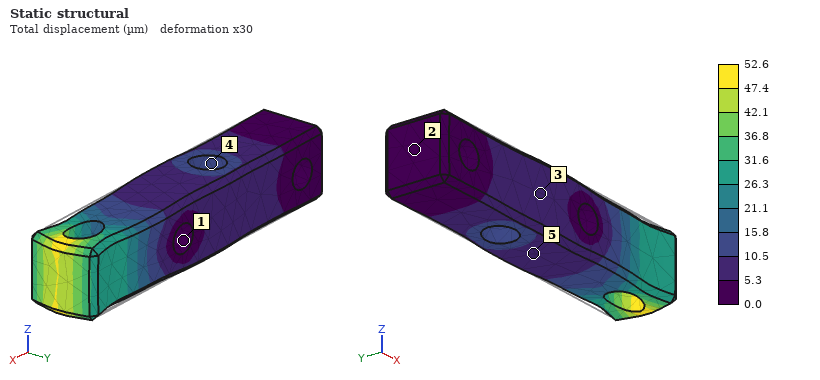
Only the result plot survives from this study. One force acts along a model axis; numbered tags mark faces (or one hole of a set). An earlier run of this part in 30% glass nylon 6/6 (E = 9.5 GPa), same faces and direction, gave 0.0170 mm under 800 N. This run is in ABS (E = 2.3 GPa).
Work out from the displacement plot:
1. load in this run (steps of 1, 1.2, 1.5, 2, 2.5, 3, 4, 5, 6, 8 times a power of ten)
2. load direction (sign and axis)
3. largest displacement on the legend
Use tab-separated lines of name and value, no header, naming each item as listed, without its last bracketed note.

load in this run	600 N
load direction	+X
largest displacement on the legend	52.6 µm
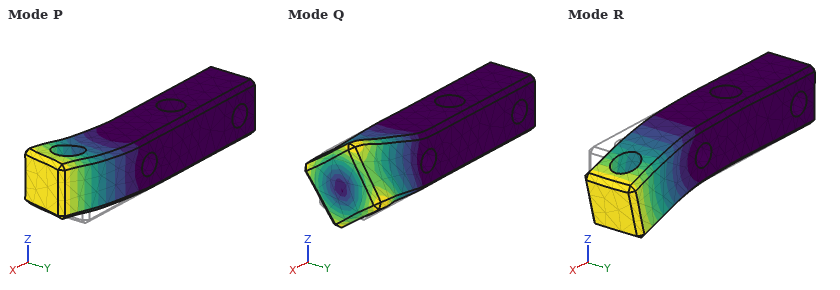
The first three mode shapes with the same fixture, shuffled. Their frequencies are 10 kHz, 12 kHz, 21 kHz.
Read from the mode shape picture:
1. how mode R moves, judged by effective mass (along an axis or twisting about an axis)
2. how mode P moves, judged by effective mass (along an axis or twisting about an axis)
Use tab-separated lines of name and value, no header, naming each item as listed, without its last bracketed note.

how mode R moves, judged by effective mass	along Z
how mode P moves, judged by effective mass	along Y
